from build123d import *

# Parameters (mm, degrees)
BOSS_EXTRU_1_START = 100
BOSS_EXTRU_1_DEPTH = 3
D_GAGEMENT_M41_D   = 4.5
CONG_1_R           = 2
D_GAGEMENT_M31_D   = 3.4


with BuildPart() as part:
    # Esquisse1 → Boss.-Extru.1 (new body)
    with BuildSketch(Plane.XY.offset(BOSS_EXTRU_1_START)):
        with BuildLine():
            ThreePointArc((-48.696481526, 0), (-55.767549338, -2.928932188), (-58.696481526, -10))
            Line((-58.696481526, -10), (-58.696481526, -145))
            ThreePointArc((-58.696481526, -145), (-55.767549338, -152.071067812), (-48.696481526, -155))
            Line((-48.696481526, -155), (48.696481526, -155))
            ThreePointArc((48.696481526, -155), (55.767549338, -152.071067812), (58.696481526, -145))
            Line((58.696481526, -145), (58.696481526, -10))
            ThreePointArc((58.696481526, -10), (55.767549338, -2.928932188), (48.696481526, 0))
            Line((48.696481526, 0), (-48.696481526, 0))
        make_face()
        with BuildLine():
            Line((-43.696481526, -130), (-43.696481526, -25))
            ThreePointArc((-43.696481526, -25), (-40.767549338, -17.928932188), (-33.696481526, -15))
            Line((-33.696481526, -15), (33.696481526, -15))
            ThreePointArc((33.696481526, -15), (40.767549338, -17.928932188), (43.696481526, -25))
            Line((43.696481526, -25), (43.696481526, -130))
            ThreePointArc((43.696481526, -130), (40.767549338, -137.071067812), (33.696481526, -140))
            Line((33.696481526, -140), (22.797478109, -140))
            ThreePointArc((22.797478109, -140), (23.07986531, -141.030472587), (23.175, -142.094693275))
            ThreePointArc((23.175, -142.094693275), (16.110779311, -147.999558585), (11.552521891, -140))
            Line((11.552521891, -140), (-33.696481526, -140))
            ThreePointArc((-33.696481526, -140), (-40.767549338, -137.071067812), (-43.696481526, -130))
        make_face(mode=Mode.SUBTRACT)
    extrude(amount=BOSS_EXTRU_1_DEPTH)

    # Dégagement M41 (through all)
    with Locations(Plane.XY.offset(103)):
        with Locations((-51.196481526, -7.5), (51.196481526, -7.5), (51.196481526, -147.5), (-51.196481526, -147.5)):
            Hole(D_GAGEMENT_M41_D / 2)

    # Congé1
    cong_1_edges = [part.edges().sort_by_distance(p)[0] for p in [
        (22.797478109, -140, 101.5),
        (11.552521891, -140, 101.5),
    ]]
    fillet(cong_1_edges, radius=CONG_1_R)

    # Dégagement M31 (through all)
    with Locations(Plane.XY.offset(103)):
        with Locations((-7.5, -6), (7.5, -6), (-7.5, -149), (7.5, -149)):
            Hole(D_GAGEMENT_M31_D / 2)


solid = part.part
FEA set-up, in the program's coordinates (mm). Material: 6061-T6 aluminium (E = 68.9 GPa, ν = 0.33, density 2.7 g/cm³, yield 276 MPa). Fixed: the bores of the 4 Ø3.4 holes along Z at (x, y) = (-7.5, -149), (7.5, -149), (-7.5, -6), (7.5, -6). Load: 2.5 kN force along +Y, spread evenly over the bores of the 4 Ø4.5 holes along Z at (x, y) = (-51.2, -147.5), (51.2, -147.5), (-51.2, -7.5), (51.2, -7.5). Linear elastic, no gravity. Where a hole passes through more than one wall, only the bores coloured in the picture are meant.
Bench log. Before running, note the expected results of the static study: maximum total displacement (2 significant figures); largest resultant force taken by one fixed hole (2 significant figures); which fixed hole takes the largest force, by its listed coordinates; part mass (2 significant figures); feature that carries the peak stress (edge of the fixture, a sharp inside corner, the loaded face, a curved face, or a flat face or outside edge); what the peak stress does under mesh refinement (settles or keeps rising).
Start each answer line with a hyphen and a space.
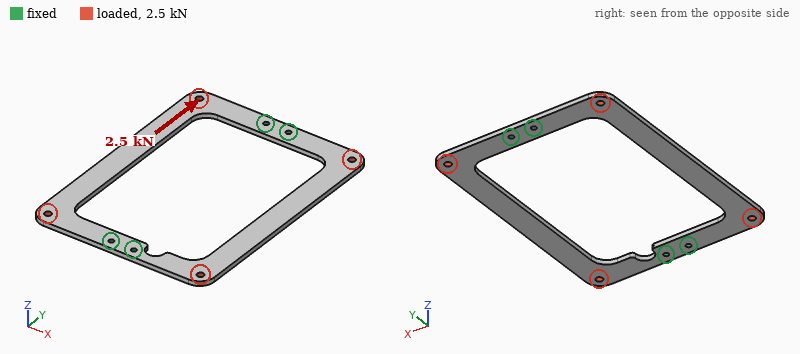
- 0.25 mm
- 1.2 kN
- (7.5, -6)
- 57 g
- edge of the fixture
- keeps rising
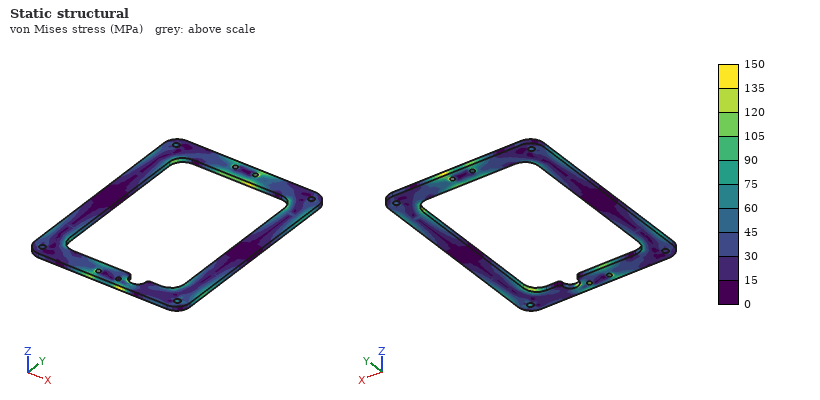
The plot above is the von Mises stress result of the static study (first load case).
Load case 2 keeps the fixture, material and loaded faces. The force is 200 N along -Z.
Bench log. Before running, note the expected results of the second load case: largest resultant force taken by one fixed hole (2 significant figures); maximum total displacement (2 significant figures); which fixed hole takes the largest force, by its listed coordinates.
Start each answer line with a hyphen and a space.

- 62 N
- 1.1 mm
- (-7.5, -149)
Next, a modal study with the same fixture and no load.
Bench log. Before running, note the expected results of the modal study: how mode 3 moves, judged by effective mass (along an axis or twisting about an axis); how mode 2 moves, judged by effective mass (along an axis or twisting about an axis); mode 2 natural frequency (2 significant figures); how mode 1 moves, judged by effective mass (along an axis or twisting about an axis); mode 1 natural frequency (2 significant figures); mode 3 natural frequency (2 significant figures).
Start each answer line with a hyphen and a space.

- twisting about X
- along Z
- 380 Hz
- along Z
- 340 Hz
- 770 Hz
